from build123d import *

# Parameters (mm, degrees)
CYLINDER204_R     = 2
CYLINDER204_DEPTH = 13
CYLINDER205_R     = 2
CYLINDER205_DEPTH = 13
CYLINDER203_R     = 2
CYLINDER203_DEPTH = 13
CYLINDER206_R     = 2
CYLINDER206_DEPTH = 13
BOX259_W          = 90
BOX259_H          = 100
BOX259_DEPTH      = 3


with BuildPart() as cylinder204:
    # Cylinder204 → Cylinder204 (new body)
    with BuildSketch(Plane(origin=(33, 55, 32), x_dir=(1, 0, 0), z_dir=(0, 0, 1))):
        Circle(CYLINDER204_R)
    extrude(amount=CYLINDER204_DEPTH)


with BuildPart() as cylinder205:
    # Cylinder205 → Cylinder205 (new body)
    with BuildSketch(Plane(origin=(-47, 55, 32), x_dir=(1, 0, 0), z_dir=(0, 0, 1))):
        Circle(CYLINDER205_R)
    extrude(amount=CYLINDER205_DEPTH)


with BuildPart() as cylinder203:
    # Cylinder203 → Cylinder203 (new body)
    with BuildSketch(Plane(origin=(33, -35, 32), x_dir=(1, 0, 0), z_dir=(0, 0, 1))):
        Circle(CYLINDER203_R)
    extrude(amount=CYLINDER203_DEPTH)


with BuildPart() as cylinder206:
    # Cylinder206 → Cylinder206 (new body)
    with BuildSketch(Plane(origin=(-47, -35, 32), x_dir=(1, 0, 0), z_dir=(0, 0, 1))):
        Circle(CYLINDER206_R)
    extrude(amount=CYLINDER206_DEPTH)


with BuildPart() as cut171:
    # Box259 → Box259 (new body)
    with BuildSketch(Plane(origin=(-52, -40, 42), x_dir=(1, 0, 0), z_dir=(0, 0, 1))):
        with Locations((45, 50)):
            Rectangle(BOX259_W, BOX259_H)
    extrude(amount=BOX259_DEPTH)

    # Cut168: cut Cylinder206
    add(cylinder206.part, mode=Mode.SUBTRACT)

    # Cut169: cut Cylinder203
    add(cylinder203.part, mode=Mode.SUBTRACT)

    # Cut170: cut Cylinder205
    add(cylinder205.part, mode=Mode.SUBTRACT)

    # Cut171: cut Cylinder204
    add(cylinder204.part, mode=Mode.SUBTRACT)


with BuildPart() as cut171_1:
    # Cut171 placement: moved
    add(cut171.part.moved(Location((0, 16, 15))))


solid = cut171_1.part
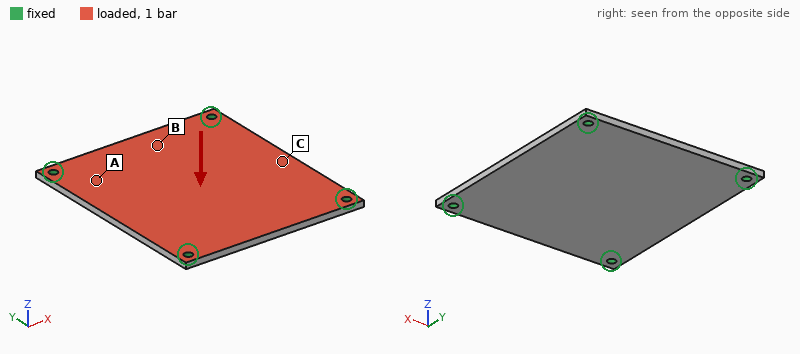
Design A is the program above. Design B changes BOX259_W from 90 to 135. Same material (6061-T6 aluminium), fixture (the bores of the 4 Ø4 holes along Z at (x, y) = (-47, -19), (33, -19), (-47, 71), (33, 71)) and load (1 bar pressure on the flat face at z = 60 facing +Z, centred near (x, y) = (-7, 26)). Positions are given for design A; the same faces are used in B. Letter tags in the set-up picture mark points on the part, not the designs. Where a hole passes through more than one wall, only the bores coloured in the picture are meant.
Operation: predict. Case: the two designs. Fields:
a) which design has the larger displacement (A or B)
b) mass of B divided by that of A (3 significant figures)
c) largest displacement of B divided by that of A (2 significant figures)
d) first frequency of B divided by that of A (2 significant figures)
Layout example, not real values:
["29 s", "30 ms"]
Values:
["A", "1.50", "0.88", "1.1"]
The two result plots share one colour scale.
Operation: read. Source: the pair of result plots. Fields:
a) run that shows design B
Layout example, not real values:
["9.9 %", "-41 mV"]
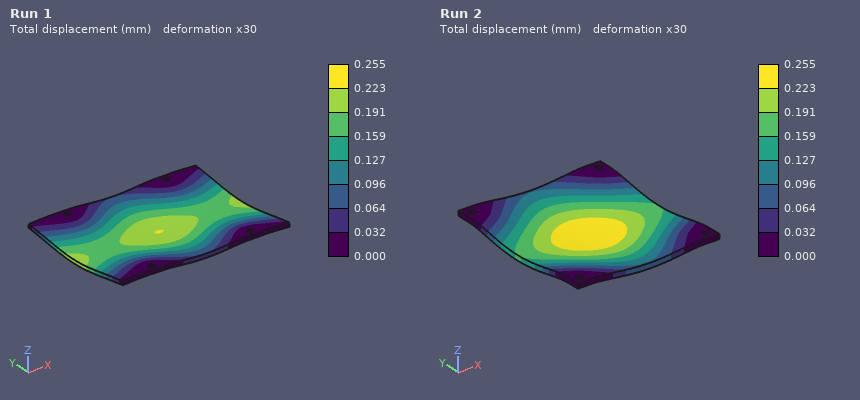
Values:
["Run 1"]
